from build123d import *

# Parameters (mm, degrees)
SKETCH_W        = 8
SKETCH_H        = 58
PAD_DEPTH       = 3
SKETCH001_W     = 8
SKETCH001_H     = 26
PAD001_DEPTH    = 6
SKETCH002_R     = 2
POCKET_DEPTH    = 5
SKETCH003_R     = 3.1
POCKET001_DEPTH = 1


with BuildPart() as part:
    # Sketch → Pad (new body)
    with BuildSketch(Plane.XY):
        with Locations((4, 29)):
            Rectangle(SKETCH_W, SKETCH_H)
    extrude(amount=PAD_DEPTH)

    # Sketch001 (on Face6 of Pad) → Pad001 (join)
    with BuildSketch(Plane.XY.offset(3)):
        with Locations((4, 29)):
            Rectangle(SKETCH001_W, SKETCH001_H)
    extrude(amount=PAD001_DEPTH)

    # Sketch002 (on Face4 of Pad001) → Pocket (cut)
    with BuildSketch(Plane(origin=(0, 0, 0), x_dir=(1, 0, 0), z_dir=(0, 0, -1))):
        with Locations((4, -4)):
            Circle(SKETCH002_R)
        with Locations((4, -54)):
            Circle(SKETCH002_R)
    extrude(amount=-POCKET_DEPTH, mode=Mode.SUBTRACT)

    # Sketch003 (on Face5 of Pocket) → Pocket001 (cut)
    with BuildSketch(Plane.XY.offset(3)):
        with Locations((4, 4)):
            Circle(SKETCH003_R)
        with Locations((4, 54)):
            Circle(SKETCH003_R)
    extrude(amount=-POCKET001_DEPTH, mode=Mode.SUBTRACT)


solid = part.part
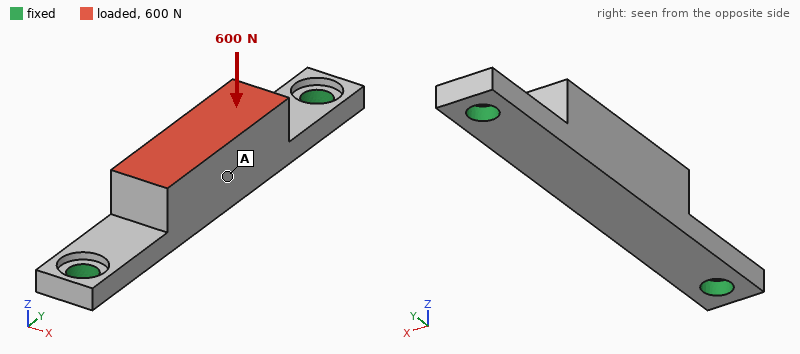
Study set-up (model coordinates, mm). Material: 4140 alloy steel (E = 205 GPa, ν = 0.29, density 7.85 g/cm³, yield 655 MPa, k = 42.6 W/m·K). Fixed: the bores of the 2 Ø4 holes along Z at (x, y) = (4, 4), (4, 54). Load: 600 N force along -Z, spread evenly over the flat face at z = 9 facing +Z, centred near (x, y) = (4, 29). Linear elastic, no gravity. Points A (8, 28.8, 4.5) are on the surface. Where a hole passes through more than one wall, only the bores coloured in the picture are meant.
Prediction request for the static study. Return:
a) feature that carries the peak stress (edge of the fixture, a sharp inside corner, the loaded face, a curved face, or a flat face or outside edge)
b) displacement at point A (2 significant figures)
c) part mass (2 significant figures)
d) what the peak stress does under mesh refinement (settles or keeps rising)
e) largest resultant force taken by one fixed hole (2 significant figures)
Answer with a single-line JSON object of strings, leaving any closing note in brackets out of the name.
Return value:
{"feature that carries the peak stress": "edge of the fixture", "displacement at point A": "21 µm", "part mass": "20 g", "what the peak stress does under mesh refinement": "keeps rising", "largest resultant force taken by one fixed hole": "510 N"}
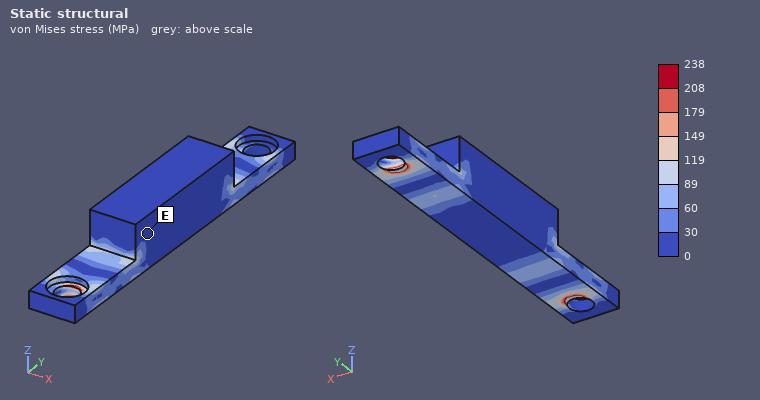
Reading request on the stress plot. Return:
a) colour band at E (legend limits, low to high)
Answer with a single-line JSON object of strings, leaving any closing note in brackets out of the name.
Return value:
{"colour band at E": "0 to 30 MPa"}
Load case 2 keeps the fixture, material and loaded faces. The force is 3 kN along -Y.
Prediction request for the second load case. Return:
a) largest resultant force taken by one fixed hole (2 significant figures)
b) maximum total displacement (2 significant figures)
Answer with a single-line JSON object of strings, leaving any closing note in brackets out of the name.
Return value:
{"largest resultant force taken by one fixed hole": "1.6 kN", "maximum total displacement": "29 µm"}
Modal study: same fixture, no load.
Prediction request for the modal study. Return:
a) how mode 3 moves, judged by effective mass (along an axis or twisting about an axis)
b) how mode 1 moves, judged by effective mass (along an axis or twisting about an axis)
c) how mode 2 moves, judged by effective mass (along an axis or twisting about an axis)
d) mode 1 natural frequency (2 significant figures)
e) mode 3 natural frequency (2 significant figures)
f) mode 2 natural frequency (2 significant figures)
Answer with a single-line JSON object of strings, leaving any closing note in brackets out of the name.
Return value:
{"how mode 3 moves, judged by effective mass": "along X", "how mode 1 moves, judged by effective mass": "along X", "how mode 2 moves, judged by effective mass": "along Z", "mode 1 natural frequency": "6500 Hz", "mode 3 natural frequency": "15 kHz", "mode 2 natural frequency": "6900 Hz"}
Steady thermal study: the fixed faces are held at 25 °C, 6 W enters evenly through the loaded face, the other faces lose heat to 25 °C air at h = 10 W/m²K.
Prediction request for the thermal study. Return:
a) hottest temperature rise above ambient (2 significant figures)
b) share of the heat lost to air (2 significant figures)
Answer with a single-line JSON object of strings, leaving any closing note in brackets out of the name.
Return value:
{"hottest temperature rise above ambient": "45 K", "share of the heat lost to air": "6.5 %"}
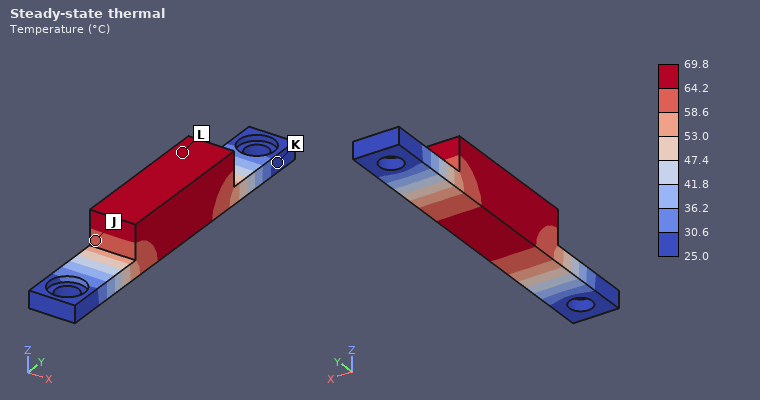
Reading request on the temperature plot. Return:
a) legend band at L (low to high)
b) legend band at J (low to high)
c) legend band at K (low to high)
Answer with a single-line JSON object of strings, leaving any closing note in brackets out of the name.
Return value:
{"legend band at L": "64.2 to 69.8 °C", "legend band at J": "58.6 to 64.2 °C", "legend band at K": "25.0 to 30.6 °C"}
